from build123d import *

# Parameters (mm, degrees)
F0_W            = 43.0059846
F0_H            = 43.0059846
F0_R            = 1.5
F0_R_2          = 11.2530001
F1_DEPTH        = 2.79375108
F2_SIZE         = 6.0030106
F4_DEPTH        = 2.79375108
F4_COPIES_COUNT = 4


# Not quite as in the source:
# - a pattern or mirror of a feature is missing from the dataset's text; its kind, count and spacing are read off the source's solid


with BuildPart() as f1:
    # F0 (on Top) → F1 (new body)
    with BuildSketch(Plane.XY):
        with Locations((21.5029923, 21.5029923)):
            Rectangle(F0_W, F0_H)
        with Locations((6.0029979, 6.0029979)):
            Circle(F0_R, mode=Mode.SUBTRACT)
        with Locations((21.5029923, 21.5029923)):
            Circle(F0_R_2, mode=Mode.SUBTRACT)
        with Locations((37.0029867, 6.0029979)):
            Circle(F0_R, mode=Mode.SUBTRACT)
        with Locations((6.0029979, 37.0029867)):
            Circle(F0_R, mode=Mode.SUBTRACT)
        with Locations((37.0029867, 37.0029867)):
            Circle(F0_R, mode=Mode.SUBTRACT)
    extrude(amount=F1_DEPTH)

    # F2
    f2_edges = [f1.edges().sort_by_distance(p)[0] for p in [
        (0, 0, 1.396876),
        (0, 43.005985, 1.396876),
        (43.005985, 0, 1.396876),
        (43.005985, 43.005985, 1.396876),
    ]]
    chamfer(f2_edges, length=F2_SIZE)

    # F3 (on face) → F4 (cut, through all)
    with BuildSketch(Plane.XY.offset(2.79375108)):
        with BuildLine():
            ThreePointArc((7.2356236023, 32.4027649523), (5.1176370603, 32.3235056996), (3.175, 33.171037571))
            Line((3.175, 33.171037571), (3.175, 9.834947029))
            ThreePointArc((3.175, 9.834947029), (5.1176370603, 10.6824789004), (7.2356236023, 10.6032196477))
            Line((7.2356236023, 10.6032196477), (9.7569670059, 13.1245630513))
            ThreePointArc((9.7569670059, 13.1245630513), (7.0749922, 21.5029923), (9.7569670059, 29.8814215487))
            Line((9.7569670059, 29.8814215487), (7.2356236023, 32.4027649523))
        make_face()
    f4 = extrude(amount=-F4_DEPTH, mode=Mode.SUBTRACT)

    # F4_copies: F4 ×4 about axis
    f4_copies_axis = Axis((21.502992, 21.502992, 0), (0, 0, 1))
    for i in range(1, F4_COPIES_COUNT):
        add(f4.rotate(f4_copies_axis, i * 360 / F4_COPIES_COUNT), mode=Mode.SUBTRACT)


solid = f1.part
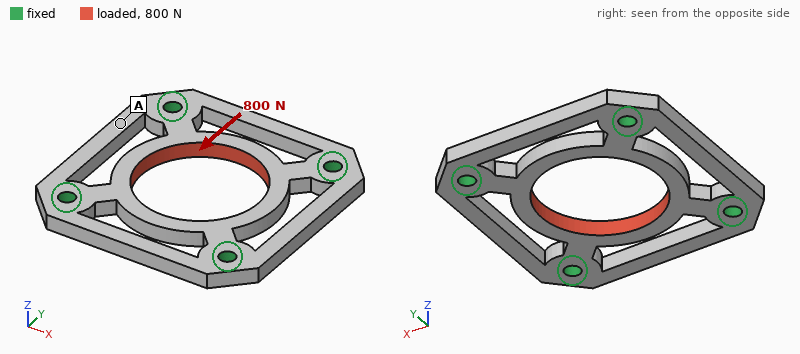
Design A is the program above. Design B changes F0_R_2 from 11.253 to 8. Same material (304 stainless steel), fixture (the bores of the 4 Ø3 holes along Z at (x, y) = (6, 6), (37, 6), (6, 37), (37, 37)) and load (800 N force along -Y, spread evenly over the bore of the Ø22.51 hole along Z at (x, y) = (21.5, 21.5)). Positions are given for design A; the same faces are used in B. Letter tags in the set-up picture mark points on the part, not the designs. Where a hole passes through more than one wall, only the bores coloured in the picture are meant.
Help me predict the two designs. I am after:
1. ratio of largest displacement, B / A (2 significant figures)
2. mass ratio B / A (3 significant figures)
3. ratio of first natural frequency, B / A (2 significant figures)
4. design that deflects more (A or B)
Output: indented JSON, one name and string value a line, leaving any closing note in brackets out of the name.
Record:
{
  "ratio of largest displacement, B / A": "0.33",
  "mass ratio B / A": "1.21",
  "ratio of first natural frequency, B / A": "0.75",
  "design that deflects more": "A"
}
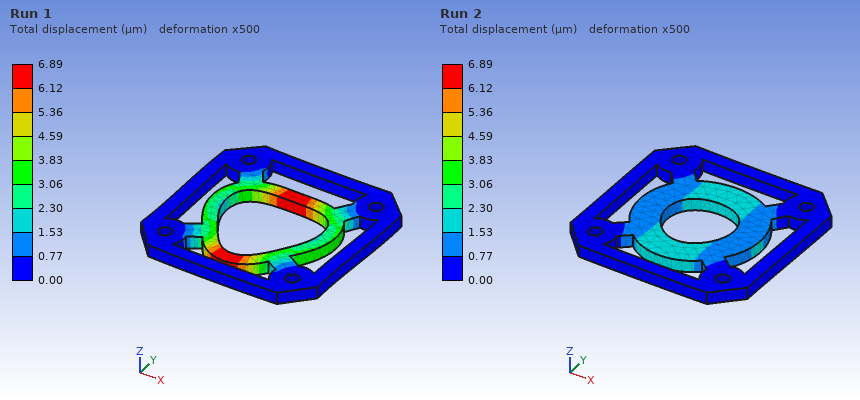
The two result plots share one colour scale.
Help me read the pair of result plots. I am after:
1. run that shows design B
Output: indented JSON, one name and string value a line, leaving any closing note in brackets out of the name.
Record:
{
  "run that shows design B": "Run 2"
}
